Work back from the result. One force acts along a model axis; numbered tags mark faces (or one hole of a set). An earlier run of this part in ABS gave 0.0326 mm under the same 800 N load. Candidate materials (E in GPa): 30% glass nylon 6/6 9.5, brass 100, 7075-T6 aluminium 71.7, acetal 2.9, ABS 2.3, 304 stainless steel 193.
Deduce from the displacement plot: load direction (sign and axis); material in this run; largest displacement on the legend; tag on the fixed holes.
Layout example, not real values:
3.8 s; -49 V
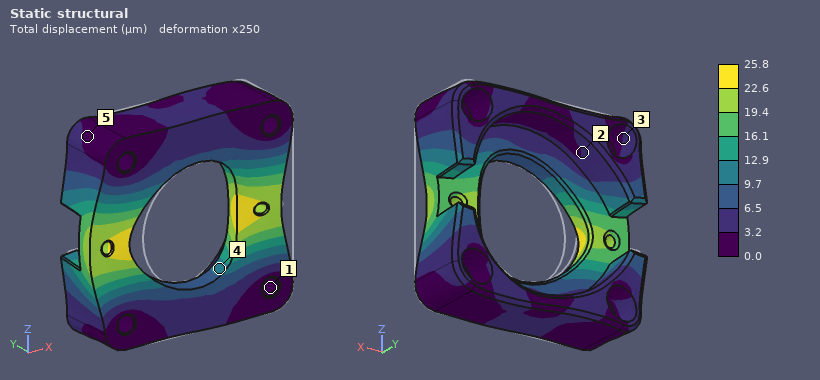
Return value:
-X; acetal; 25.8 µm; 1
